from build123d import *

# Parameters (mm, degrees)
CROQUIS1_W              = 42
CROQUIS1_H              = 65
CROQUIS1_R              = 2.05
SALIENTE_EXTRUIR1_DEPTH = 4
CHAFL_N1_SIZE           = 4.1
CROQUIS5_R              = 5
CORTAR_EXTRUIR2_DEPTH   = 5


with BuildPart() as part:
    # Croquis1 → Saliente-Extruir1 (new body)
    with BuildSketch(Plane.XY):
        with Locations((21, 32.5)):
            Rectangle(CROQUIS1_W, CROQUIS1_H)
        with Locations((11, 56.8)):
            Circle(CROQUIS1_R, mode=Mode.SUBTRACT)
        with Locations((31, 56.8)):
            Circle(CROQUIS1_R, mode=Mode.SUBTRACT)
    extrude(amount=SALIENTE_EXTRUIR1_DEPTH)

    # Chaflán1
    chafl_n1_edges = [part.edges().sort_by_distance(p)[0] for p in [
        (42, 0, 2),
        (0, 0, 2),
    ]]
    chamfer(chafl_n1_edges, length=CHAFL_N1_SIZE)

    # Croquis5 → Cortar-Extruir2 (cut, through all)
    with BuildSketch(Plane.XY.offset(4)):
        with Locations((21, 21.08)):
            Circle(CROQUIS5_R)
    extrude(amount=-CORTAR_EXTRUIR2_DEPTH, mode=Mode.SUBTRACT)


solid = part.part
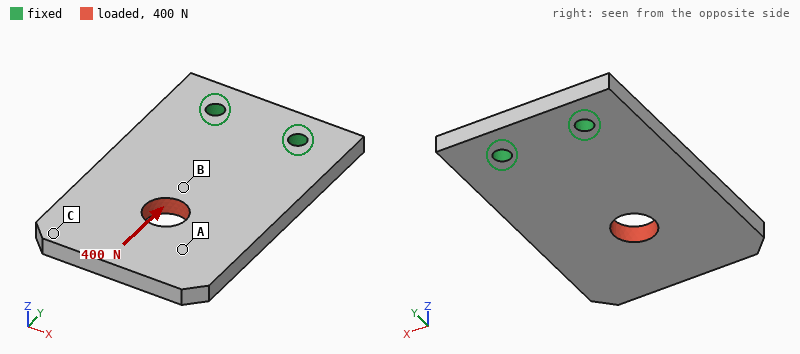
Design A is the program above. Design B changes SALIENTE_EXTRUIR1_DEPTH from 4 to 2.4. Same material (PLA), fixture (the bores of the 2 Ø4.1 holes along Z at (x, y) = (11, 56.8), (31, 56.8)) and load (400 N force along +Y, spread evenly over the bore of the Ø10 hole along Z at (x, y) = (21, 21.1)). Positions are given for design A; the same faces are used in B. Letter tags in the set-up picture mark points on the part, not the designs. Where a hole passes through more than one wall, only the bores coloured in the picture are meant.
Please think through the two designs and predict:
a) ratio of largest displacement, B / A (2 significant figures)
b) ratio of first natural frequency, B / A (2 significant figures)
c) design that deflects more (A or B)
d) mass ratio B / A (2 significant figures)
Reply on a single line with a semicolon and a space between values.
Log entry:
1.7; 0.61; B; 0.60
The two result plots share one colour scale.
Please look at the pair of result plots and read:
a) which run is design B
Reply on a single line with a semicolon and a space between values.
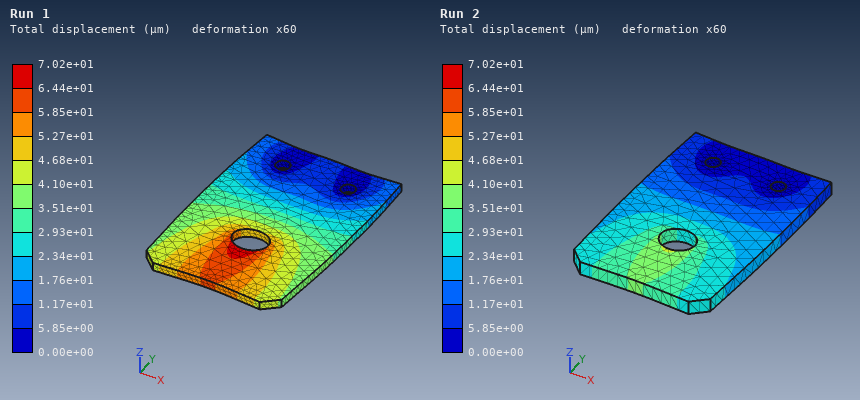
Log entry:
Run 1
